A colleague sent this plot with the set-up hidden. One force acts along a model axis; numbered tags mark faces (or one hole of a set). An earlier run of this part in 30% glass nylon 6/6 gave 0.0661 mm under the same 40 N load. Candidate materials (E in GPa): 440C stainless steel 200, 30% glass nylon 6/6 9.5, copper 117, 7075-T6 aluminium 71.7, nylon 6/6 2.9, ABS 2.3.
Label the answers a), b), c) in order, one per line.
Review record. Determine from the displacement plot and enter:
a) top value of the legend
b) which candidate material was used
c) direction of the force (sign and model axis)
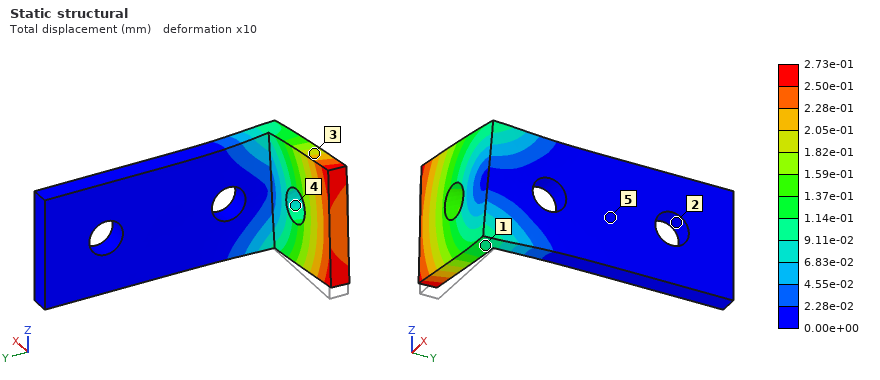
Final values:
a) 2.73e-01 mm
b) ABS
c) +Z
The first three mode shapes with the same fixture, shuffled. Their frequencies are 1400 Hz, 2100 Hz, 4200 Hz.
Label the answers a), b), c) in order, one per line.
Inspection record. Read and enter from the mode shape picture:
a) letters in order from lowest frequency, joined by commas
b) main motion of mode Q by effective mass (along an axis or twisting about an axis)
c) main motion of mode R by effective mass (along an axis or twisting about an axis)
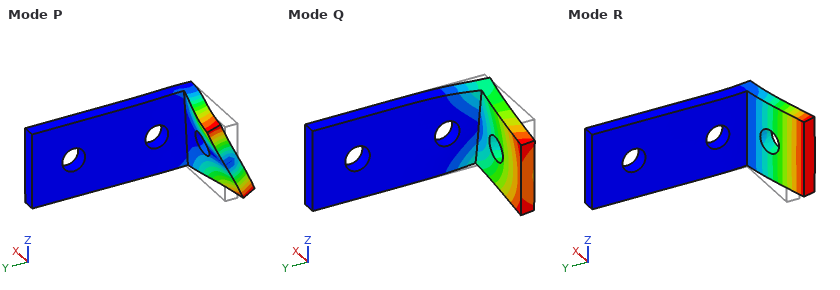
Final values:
a) R, Q, P
b) along Z
c) along Y
